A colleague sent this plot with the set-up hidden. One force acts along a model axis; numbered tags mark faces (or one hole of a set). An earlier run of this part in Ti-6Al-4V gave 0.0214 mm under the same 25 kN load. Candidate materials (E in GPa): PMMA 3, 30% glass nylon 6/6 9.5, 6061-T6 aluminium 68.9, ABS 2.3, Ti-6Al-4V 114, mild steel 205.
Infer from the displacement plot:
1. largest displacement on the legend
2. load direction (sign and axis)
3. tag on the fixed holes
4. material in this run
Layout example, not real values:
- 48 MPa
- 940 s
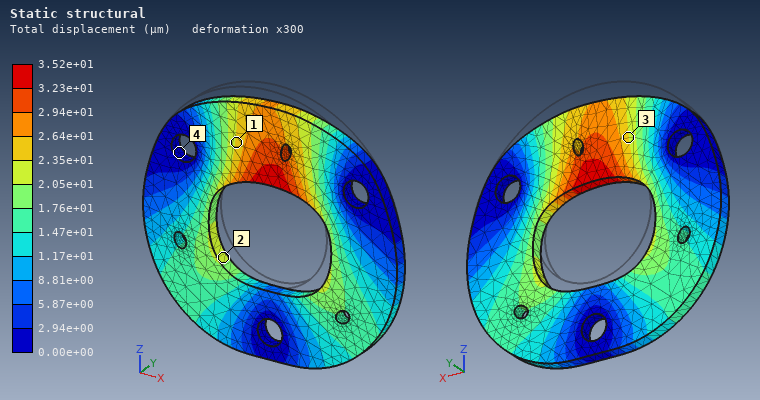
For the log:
- 3.52e+01 µm
- -Z
- 4
- 6061-T6 aluminium
